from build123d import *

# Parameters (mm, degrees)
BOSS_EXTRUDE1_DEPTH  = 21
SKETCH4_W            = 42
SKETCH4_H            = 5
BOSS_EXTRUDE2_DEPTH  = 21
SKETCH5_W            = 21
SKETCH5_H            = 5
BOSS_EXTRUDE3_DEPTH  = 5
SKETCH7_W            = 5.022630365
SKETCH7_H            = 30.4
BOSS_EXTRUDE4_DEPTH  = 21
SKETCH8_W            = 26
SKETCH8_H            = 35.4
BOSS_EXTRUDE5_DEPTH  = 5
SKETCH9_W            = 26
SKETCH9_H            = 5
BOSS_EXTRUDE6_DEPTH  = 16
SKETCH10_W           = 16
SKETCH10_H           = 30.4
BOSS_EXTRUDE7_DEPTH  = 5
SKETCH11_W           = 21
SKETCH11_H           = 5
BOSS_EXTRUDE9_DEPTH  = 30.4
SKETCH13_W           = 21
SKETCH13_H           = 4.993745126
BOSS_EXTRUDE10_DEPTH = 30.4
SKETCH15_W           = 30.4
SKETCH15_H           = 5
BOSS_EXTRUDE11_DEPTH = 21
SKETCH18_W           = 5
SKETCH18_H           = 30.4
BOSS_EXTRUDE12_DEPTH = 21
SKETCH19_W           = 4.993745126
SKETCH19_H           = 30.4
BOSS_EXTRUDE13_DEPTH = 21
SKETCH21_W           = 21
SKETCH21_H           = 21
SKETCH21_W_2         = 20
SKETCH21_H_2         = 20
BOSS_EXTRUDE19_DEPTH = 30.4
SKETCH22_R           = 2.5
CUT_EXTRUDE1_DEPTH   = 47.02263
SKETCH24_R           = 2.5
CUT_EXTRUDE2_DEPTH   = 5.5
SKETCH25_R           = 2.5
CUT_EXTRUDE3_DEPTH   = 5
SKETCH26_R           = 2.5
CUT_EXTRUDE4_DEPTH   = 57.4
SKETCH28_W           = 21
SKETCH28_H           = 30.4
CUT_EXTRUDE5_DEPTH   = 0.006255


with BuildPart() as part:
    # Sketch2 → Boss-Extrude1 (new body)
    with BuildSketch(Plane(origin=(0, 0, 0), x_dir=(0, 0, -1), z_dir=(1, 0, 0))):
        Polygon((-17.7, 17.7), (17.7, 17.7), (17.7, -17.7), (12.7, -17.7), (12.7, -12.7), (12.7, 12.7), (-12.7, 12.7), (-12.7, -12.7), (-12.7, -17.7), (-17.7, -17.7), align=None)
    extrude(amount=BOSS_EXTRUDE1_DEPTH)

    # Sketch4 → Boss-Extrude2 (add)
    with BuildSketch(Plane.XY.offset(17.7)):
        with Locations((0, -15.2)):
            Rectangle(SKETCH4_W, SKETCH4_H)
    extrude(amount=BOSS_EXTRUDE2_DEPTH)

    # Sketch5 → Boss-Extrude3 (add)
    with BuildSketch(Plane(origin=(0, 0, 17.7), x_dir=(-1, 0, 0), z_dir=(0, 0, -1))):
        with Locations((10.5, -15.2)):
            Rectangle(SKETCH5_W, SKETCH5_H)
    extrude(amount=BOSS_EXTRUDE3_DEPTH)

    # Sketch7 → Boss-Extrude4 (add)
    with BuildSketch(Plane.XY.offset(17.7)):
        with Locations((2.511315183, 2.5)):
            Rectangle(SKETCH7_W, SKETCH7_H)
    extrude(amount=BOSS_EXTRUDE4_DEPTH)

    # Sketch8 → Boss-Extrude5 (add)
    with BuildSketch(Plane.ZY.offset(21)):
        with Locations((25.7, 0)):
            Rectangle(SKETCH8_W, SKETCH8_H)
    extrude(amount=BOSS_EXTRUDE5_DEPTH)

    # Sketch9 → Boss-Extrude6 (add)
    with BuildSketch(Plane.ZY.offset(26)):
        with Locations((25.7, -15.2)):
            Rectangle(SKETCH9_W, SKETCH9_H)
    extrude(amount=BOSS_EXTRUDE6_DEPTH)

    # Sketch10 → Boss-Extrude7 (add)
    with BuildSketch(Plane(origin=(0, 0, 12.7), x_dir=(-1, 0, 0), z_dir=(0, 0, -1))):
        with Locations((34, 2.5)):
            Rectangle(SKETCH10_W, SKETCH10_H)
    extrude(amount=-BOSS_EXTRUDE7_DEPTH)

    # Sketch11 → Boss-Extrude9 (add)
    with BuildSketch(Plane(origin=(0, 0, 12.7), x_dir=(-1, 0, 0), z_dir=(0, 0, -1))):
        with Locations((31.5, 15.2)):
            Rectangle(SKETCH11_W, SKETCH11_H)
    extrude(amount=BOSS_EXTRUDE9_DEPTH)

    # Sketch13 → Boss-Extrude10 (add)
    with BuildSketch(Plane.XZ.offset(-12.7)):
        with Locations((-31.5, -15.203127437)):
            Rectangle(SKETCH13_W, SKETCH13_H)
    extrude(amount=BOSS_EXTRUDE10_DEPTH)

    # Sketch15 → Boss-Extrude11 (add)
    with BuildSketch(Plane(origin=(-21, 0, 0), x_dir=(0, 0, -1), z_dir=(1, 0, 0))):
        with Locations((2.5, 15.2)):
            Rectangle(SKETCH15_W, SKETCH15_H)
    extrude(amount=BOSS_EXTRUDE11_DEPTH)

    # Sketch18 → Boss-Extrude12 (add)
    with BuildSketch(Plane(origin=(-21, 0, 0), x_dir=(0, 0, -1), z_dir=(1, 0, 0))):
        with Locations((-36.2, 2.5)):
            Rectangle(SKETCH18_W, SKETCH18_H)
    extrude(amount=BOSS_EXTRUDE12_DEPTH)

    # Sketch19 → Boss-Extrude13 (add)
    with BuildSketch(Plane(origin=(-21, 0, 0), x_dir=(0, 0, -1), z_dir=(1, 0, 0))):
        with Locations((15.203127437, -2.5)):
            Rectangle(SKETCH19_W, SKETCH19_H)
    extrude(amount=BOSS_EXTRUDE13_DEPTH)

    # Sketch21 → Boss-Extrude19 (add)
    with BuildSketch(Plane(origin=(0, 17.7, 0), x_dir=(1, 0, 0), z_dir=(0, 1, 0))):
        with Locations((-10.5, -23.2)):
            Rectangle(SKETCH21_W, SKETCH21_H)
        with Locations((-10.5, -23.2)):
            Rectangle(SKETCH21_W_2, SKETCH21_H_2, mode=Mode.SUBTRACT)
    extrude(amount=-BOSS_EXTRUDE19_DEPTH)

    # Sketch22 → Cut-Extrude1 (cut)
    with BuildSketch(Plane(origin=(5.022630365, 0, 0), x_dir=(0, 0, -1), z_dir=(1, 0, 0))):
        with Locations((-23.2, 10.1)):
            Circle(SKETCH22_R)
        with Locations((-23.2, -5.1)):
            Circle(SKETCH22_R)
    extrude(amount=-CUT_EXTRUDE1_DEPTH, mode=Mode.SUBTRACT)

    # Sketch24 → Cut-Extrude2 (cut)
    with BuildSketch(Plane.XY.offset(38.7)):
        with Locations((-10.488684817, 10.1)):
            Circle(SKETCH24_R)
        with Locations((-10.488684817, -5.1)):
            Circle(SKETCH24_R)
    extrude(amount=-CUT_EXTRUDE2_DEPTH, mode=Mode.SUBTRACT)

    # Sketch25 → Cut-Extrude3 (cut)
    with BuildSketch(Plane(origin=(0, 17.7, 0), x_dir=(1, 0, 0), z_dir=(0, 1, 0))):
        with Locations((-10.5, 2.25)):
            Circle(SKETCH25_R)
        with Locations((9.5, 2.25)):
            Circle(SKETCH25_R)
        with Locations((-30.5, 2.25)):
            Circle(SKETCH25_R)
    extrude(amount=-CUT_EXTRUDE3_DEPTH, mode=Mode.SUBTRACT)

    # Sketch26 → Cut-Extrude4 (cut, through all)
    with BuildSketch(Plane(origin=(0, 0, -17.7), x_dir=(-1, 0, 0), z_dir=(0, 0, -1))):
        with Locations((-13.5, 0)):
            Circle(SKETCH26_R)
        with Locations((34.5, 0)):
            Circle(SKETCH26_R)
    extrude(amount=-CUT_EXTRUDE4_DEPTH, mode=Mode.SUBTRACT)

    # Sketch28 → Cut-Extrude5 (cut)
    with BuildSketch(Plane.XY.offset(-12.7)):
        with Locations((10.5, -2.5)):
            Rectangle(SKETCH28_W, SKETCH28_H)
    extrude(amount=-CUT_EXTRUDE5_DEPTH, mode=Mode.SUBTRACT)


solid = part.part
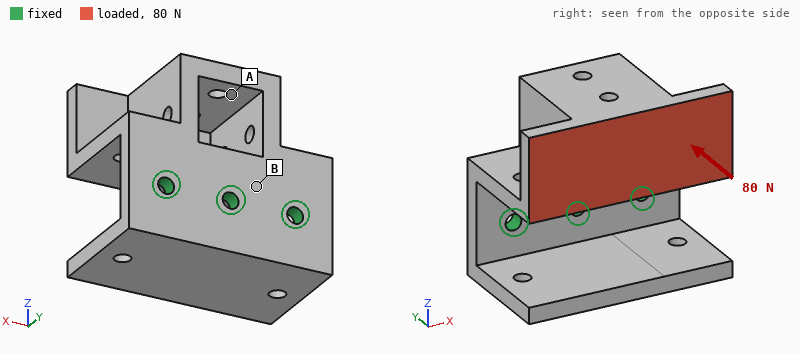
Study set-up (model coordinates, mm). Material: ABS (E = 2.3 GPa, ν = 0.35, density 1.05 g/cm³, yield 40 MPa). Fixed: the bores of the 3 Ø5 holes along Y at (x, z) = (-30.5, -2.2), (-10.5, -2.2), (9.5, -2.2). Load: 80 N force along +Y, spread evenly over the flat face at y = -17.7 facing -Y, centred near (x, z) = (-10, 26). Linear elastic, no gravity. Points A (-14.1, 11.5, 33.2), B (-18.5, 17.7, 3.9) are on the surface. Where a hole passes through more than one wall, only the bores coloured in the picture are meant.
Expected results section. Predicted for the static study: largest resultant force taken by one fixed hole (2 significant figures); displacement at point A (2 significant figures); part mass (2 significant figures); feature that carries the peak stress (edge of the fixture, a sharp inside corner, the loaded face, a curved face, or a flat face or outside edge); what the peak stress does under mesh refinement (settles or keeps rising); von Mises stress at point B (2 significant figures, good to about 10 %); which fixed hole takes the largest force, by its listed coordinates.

31 N
0.55 mm
45 g
edge of the fixture
keeps rising
4.9 MPa
(-10.5, -2.2)
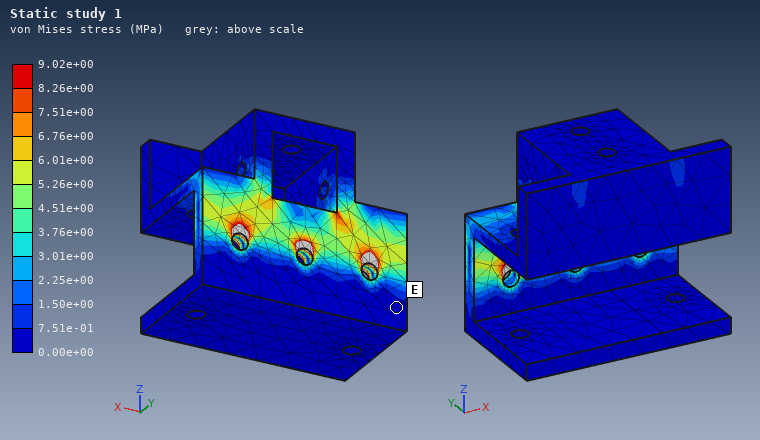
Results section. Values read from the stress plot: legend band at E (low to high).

0.00e+00 to 7.51e-01 MPa
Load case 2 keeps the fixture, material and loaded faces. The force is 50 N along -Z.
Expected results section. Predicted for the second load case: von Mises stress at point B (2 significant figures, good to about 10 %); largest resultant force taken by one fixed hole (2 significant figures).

4.6 MPa
24 N
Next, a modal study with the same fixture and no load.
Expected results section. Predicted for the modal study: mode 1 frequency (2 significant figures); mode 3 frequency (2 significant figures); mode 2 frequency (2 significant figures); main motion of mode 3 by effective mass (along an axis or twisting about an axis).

290 Hz
890 Hz
730 Hz
along X
